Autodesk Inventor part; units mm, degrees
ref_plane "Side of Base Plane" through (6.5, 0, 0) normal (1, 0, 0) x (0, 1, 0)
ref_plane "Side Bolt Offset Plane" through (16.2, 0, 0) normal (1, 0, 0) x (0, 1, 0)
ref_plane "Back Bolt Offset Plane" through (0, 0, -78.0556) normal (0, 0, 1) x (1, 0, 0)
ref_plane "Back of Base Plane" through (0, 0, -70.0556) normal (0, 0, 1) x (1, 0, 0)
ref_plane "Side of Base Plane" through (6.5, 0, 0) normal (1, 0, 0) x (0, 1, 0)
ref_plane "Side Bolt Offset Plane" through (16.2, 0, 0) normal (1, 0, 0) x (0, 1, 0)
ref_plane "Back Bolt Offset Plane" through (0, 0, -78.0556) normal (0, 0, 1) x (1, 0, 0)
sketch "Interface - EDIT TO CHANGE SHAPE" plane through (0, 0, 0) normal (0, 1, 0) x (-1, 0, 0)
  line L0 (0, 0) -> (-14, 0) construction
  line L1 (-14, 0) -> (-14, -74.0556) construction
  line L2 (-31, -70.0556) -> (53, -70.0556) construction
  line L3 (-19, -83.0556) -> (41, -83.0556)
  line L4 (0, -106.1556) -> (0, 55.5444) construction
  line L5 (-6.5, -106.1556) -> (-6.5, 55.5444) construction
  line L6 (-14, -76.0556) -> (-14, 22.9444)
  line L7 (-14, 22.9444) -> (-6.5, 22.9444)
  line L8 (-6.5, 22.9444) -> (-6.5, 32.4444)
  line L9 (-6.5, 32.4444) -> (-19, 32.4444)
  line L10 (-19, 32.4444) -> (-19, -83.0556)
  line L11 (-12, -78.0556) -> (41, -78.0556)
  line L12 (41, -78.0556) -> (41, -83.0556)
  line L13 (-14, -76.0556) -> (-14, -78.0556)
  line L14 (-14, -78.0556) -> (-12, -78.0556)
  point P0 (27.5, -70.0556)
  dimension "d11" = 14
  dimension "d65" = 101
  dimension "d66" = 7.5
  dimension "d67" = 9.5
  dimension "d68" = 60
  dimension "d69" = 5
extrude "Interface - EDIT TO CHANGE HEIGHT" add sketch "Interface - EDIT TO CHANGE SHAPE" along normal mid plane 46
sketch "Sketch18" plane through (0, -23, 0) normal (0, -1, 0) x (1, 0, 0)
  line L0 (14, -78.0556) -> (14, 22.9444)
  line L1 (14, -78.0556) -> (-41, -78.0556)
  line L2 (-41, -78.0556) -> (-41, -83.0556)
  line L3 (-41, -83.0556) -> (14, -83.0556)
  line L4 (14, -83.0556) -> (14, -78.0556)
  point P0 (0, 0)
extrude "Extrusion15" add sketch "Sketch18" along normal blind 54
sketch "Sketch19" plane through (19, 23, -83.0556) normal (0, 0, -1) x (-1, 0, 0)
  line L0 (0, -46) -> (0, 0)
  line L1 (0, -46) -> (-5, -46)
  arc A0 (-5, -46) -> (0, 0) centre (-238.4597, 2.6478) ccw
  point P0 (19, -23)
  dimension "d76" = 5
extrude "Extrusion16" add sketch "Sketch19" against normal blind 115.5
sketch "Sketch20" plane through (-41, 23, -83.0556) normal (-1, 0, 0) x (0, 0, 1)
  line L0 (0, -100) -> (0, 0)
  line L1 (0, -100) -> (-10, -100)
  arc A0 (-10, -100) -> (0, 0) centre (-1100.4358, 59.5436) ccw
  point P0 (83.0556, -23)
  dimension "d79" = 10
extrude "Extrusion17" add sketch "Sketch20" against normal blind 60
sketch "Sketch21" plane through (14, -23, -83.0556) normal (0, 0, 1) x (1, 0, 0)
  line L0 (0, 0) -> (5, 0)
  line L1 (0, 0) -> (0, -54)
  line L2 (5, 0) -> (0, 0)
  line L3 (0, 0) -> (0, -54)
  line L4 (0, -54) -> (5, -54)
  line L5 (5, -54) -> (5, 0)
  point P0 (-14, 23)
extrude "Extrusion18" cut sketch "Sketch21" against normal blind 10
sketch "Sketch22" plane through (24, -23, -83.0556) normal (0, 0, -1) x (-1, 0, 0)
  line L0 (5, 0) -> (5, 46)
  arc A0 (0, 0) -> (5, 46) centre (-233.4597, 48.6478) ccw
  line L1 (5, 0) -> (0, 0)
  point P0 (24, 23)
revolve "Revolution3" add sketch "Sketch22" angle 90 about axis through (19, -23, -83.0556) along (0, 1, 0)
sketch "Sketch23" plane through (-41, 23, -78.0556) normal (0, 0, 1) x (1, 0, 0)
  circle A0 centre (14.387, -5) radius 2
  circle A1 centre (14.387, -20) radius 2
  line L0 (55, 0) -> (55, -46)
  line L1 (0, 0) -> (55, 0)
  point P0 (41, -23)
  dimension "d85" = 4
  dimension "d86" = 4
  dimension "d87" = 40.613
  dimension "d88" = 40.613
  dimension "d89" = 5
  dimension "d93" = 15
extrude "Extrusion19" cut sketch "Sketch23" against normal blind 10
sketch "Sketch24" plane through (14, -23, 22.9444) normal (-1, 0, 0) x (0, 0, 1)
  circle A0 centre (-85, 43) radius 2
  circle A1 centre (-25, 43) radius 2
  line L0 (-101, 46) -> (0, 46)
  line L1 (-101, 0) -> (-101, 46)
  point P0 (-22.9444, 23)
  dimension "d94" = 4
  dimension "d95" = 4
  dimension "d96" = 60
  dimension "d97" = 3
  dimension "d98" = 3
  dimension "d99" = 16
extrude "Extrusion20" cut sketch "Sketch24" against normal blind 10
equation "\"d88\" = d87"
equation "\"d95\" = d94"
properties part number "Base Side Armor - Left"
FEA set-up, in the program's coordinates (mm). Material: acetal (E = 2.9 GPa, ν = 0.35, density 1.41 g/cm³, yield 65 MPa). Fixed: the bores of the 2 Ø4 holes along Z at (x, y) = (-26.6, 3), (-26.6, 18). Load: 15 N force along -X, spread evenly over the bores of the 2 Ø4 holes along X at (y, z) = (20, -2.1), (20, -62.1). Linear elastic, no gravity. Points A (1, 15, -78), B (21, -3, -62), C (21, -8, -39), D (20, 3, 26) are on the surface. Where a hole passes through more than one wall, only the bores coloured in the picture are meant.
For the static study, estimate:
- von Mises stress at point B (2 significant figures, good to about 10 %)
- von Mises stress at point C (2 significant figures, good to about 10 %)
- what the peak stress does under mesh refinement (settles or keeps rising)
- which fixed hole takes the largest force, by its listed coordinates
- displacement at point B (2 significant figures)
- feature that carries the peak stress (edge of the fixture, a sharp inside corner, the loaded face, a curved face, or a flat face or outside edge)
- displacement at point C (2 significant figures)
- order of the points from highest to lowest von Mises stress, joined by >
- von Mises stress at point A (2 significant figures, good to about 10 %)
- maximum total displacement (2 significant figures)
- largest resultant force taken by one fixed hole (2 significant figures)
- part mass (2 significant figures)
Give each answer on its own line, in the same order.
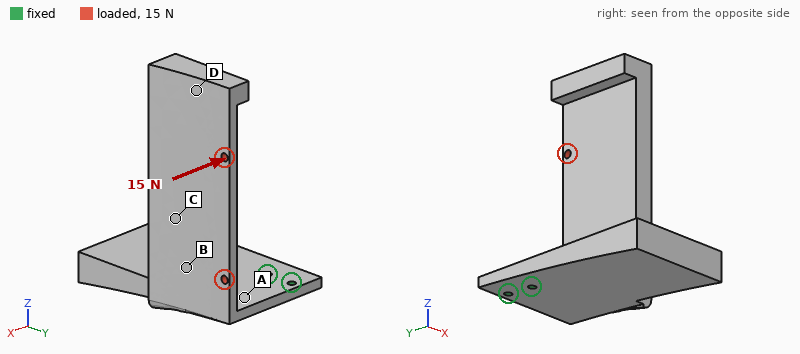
1.2 MPa
0.94 MPa
keeps rising
(-26.6, 18)
0.32 mm
edge of the fixture
0.53 mm
A > B > C > D
1.7 MPa
1.6 mm
16 N
130 g
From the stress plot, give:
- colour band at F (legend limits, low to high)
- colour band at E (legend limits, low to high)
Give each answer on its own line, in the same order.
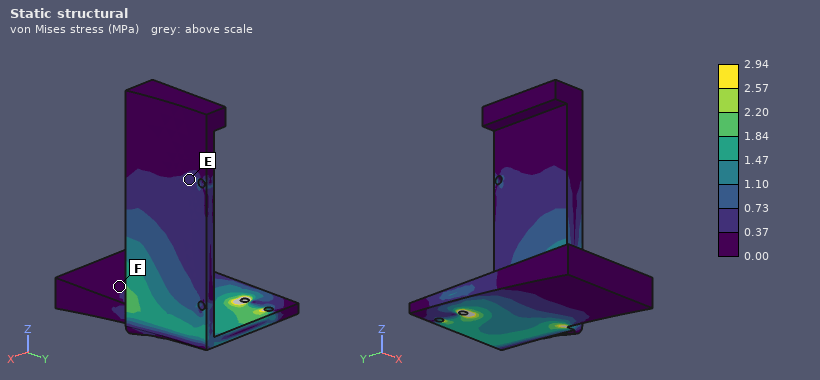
0.00 to 0.37 MPa
0.37 to 0.73 MPa
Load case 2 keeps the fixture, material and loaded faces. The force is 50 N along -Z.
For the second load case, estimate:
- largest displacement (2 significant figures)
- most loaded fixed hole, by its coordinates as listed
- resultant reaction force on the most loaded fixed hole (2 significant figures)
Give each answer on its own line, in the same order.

2.0 mm
(-26.6, 18)
38 N
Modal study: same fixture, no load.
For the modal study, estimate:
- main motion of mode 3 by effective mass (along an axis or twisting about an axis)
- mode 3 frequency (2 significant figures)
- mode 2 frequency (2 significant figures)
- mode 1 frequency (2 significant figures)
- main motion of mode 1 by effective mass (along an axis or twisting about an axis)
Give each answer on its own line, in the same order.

along Z
240 Hz
93 Hz
69 Hz
along X
